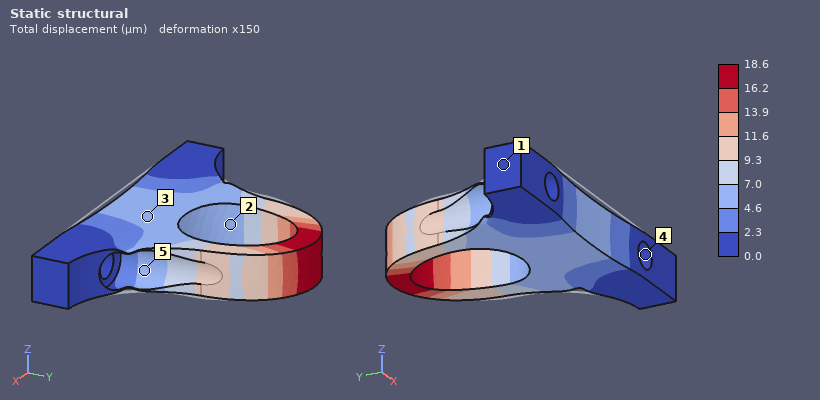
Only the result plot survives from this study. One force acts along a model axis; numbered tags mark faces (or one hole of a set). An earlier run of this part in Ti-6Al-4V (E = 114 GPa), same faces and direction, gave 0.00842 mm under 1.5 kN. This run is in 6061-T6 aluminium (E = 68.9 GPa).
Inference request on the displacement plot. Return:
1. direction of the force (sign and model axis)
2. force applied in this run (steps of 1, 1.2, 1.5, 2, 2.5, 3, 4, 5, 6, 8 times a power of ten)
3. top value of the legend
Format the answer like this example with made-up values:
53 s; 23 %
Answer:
+Y; 2 kN; 18.6 µm
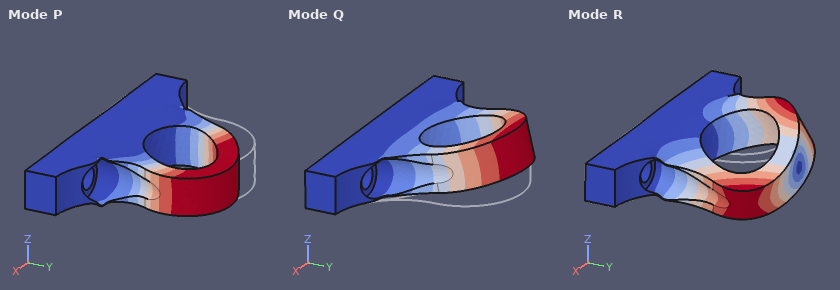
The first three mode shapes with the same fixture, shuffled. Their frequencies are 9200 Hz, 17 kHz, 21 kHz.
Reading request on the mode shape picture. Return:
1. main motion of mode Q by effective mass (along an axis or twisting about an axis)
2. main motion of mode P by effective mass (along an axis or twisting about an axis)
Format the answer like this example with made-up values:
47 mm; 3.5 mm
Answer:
along Z; along X
